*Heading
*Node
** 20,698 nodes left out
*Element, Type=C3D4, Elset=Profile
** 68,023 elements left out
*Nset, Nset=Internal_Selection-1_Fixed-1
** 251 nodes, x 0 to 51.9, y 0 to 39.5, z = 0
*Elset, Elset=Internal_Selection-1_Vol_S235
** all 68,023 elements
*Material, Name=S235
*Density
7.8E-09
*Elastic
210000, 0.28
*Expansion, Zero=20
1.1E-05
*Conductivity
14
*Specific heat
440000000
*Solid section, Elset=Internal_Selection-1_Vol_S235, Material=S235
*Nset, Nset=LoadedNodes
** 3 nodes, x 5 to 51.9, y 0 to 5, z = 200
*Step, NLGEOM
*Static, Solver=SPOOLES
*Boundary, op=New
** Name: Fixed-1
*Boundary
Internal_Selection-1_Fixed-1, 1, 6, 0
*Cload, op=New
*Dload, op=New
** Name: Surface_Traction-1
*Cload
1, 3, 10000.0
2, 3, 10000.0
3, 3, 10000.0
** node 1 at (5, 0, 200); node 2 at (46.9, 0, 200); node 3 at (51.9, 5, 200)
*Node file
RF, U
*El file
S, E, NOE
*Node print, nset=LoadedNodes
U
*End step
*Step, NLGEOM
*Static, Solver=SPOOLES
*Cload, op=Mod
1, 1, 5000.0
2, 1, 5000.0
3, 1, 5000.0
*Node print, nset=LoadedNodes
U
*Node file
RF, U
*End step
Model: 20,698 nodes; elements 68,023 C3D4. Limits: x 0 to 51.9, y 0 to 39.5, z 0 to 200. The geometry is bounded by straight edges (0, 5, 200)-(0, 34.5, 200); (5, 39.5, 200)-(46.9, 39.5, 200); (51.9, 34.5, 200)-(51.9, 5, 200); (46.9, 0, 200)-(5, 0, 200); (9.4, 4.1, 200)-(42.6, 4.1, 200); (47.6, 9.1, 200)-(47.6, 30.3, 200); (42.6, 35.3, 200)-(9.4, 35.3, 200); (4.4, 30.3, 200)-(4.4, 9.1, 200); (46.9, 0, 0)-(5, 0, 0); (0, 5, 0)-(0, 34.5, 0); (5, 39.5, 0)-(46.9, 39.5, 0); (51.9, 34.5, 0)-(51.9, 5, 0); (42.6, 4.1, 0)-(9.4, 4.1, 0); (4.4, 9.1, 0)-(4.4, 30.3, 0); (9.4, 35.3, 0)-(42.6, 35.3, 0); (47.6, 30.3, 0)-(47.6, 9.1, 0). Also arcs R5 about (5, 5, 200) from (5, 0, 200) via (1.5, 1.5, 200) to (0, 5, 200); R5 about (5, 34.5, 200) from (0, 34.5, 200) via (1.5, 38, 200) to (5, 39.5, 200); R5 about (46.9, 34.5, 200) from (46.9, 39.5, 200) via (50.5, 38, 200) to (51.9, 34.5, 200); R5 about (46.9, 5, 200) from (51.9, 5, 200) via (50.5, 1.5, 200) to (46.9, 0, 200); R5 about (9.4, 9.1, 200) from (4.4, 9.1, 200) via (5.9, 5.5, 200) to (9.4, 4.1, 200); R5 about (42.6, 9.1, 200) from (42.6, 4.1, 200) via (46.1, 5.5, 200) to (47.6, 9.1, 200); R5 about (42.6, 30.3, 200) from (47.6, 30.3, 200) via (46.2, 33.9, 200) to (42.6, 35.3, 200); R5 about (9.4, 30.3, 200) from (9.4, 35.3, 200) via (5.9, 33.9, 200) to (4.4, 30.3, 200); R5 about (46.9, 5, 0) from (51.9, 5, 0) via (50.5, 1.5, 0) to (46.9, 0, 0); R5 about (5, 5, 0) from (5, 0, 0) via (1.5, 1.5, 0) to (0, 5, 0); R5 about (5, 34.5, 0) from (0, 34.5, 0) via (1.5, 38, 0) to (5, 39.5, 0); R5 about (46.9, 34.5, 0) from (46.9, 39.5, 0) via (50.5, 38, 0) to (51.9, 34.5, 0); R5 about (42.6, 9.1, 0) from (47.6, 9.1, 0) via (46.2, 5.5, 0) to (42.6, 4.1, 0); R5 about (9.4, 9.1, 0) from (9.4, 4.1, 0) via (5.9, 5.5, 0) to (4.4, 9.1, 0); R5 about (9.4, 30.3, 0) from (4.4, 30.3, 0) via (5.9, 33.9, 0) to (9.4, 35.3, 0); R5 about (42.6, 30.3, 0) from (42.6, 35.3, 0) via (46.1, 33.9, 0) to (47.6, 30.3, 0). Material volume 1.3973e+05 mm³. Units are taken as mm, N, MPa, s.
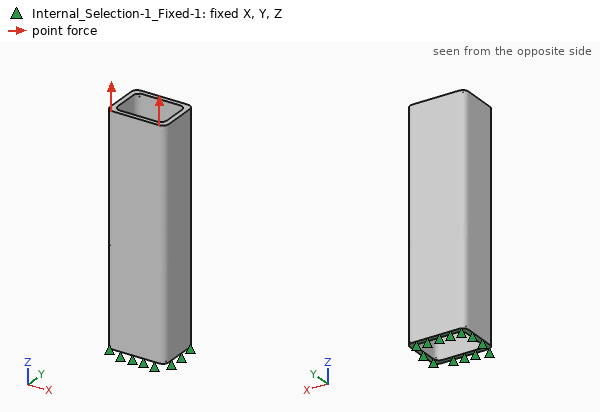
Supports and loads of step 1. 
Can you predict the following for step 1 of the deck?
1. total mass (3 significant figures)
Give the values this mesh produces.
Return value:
1.09 kg
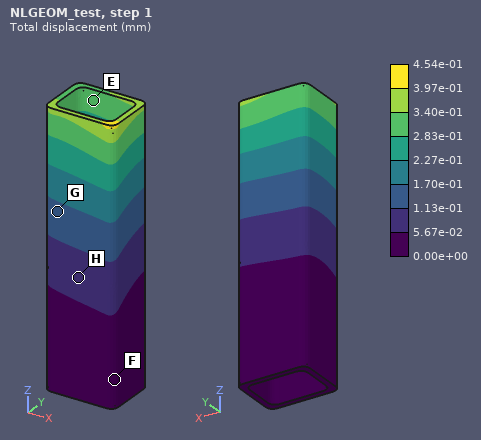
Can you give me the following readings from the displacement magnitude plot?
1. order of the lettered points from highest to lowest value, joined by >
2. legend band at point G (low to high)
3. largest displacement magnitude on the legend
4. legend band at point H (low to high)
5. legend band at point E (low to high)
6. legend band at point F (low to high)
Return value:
E > G > H > F
1.13e-01 to 1.70e-01 mm
4.54e-01 mm
5.67e-02 to 1.13e-01 mm
2.83e-01 to 3.40e-01 mm
0.00e+00 to 5.67e-02 mm
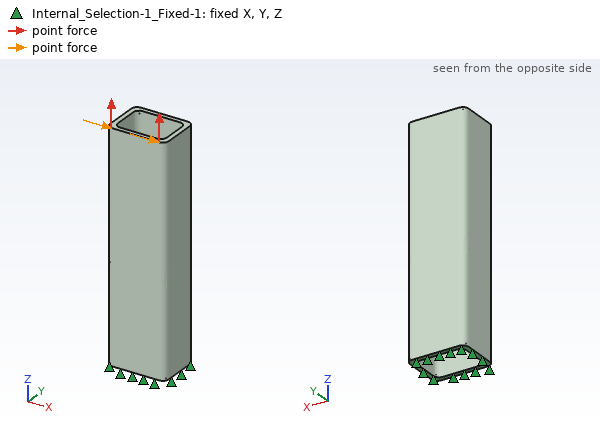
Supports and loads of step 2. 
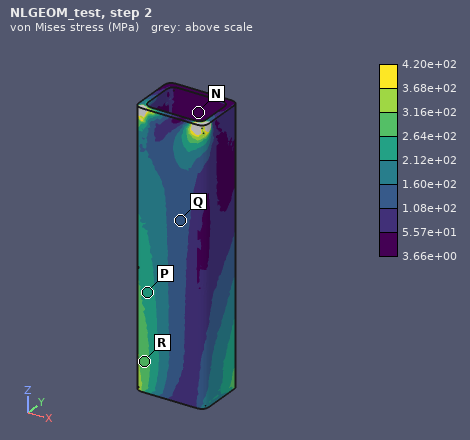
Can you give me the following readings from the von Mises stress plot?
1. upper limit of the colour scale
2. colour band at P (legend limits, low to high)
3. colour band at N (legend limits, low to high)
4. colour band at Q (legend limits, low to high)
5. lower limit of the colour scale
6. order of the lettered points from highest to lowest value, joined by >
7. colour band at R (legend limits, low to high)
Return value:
4.20e+02 MPa
2.12e+02 to 2.64e+02 MPa
3.66e+00 to 5.57e+01 MPa
1.08e+02 to 1.60e+02 MPa
3.66e+00 MPa
R > P > Q > N
2.64e+02 to 3.16e+02 MPa
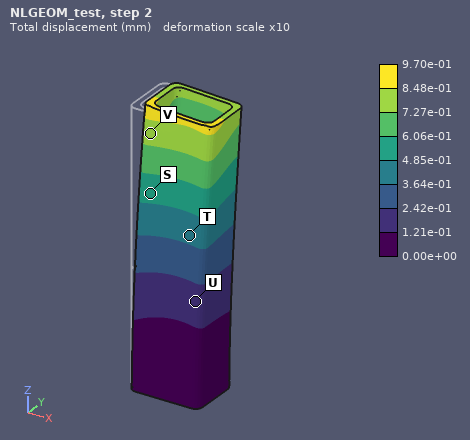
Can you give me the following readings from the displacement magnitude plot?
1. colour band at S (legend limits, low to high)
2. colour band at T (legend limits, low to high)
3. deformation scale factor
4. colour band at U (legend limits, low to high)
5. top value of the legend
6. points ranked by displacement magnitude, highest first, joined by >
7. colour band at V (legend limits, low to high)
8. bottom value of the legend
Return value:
4.85e-01 to 6.06e-01 mm
3.64e-01 to 4.85e-01 mm
10
1.21e-01 to 2.42e-01 mm
9.70e-01 mm
V > S > T > U
7.27e-01 to 8.48e-01 mm
0.00e+00 mm
